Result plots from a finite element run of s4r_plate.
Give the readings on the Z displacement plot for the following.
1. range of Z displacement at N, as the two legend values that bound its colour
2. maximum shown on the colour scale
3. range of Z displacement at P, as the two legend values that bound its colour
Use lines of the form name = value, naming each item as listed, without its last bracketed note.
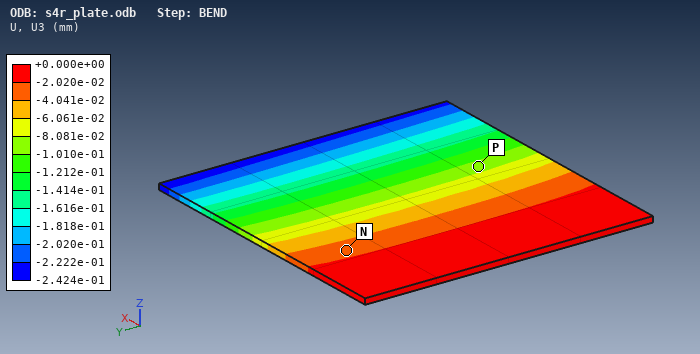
range of Z displacement at N, as the two legend values that bound its colour = -4.041e-02 to -2.020e-02 mm
maximum shown on the colour scale = +0.000e+00 mm
range of Z displacement at P, as the two legend values that bound its colour = -1.010e-01 to -8.081e-02 mm
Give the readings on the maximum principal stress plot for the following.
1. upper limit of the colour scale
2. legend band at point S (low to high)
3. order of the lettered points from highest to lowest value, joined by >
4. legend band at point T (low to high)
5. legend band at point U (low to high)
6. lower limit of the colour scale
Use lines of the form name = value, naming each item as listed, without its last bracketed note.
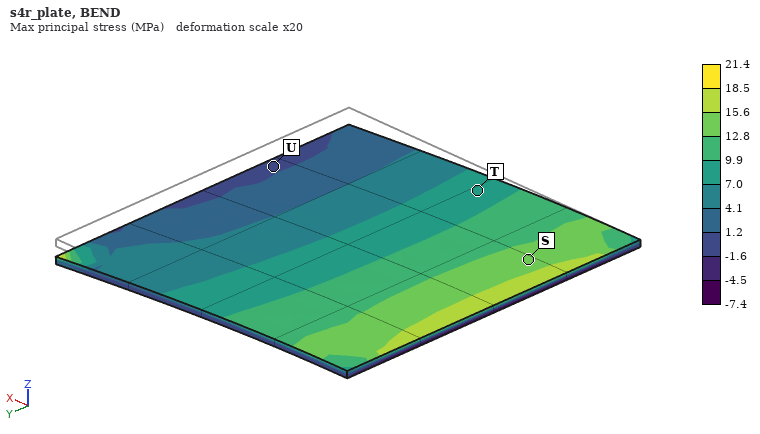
upper limit of the colour scale = 21.4 MPa
legend band at point S = 12.8 to 15.6 MPa
order of the lettered points from highest to lowest value, joined by > = S > T > U
legend band at point T = 7.0 to 9.9 MPa
legend band at point U = -1.6 to 1.2 MPa
lower limit of the colour scale = -7.4 MPa
